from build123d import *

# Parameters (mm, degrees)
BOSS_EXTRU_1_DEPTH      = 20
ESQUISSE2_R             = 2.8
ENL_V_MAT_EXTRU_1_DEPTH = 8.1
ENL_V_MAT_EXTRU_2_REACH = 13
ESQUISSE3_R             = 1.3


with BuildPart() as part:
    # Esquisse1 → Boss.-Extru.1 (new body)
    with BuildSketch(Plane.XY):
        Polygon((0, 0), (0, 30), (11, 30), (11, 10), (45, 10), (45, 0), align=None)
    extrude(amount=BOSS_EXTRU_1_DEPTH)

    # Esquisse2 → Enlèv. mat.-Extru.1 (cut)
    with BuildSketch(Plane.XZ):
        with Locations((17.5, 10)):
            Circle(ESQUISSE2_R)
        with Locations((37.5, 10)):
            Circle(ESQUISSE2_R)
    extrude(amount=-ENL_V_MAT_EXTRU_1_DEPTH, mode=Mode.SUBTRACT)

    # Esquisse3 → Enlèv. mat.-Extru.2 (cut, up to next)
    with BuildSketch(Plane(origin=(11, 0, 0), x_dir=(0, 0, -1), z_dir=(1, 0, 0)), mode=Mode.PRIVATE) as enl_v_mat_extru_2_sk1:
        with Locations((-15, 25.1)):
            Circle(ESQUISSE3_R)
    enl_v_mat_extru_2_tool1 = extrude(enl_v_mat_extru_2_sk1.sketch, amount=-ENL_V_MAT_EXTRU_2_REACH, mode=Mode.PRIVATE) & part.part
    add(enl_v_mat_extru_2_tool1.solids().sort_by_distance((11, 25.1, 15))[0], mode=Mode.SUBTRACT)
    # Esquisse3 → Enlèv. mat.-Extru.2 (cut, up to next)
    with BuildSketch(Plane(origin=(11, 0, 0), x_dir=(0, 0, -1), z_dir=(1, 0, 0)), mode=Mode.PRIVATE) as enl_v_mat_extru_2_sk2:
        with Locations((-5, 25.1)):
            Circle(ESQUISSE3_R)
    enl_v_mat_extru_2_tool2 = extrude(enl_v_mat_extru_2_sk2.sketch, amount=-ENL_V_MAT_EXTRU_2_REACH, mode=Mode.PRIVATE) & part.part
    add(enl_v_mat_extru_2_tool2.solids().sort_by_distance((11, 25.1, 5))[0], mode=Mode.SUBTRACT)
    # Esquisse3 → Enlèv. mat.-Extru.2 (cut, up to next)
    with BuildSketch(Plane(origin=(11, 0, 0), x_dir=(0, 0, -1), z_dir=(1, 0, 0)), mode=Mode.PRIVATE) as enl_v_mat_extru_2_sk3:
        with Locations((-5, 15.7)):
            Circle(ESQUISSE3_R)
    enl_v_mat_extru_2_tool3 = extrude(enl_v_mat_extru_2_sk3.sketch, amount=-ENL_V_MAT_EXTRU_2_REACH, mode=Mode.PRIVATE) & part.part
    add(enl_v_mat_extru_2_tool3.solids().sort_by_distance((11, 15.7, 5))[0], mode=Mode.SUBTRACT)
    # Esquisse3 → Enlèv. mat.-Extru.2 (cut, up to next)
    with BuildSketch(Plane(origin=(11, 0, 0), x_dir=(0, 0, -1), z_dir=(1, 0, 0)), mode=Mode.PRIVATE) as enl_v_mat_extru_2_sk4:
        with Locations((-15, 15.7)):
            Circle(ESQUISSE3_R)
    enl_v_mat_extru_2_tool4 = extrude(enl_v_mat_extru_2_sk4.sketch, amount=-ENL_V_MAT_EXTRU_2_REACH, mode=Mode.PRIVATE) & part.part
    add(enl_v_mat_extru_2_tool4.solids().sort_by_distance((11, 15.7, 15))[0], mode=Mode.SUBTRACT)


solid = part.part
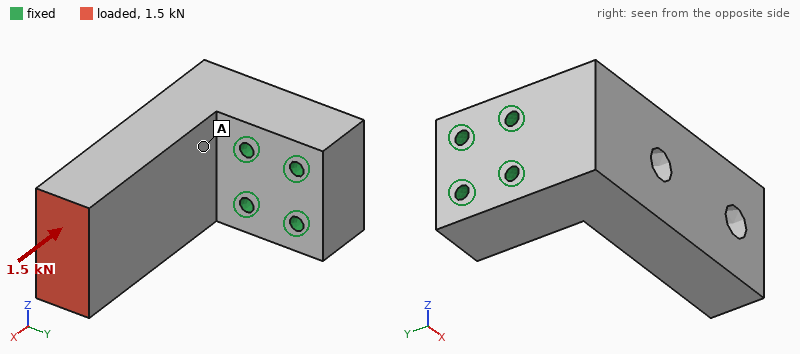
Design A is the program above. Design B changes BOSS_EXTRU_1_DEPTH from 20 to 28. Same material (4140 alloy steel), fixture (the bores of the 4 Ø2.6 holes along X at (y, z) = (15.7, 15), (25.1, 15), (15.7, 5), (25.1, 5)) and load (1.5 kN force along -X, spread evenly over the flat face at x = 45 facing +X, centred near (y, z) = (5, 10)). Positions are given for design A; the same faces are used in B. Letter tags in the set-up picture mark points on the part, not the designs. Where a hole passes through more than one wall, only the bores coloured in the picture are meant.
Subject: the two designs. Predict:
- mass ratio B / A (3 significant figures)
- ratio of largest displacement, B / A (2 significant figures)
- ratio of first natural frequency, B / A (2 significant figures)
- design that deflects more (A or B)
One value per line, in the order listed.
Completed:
1.42
0.85
0.97
A
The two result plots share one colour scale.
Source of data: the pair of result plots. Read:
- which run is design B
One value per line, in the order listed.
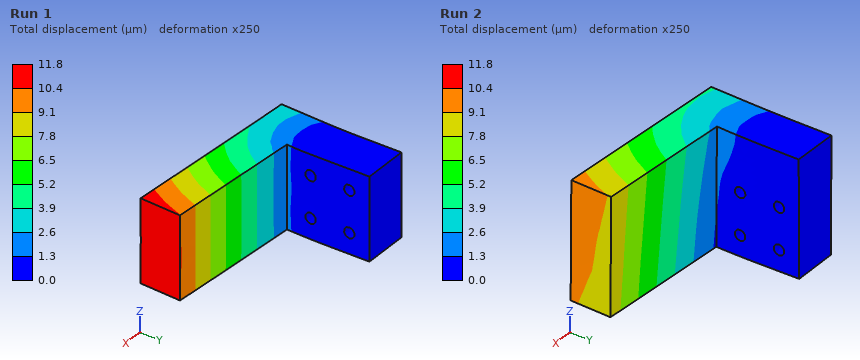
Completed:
Run 2
